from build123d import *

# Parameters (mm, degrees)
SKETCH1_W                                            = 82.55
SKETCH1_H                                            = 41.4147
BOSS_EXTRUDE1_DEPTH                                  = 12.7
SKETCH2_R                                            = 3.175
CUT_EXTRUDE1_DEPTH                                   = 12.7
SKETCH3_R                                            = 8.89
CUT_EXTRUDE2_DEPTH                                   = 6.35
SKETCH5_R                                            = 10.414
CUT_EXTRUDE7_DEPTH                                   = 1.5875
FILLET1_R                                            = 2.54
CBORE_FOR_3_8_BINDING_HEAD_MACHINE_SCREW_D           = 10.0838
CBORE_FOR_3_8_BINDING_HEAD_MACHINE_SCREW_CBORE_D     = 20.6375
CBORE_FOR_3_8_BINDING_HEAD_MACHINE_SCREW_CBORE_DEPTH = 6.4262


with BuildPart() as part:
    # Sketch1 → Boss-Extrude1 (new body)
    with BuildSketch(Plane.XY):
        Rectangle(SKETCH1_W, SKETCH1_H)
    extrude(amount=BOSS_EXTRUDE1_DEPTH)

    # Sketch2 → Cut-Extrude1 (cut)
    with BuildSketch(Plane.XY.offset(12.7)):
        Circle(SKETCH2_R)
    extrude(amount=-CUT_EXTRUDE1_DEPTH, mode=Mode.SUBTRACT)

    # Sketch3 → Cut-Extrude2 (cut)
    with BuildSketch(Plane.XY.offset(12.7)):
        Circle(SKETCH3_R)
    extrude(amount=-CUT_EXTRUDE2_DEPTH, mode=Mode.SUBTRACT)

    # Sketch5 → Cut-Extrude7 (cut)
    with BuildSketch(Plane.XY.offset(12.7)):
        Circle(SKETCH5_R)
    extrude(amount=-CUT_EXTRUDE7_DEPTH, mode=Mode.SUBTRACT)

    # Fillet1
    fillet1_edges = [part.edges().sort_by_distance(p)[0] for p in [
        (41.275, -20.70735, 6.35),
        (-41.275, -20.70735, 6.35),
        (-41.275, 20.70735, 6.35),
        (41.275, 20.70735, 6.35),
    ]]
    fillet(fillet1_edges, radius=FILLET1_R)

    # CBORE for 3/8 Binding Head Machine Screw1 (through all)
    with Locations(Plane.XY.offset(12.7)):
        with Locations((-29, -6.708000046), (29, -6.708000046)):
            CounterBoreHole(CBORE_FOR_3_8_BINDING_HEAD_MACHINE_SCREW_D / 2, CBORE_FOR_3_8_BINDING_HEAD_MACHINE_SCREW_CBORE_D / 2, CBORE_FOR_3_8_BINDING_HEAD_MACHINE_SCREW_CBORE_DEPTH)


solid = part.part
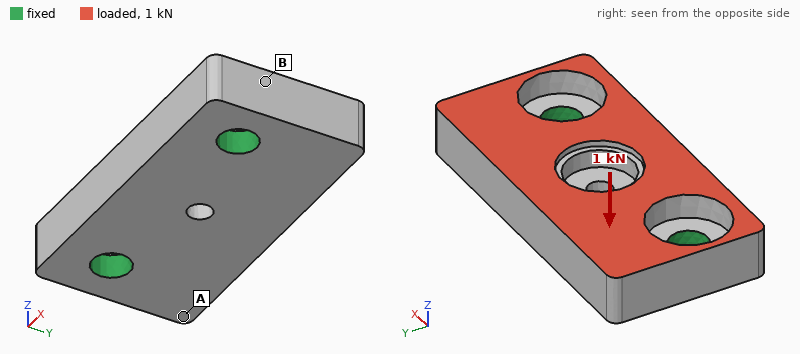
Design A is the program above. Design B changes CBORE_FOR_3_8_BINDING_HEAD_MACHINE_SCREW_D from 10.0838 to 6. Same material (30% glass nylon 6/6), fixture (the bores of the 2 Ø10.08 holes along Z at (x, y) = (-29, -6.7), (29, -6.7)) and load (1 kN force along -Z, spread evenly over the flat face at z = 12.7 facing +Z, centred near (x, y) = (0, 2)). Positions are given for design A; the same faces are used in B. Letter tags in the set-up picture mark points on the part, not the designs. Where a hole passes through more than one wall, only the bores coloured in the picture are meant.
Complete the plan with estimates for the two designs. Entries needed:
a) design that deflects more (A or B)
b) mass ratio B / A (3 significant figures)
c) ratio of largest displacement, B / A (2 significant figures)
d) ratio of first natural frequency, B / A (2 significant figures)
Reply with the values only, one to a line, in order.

B
1.02
1.6
0.75
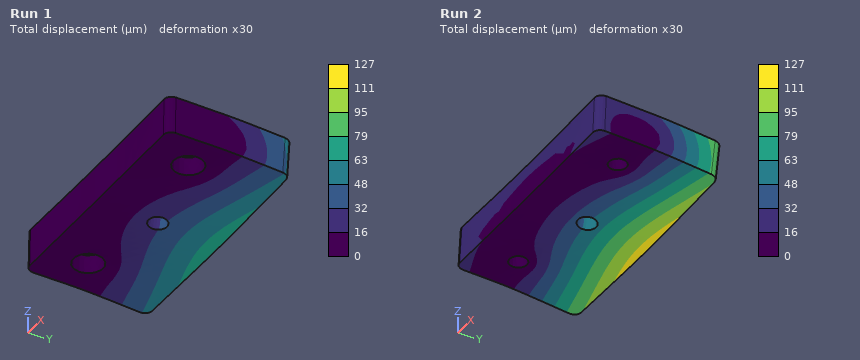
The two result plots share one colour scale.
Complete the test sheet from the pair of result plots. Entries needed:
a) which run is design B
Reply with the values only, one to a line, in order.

Run 2
